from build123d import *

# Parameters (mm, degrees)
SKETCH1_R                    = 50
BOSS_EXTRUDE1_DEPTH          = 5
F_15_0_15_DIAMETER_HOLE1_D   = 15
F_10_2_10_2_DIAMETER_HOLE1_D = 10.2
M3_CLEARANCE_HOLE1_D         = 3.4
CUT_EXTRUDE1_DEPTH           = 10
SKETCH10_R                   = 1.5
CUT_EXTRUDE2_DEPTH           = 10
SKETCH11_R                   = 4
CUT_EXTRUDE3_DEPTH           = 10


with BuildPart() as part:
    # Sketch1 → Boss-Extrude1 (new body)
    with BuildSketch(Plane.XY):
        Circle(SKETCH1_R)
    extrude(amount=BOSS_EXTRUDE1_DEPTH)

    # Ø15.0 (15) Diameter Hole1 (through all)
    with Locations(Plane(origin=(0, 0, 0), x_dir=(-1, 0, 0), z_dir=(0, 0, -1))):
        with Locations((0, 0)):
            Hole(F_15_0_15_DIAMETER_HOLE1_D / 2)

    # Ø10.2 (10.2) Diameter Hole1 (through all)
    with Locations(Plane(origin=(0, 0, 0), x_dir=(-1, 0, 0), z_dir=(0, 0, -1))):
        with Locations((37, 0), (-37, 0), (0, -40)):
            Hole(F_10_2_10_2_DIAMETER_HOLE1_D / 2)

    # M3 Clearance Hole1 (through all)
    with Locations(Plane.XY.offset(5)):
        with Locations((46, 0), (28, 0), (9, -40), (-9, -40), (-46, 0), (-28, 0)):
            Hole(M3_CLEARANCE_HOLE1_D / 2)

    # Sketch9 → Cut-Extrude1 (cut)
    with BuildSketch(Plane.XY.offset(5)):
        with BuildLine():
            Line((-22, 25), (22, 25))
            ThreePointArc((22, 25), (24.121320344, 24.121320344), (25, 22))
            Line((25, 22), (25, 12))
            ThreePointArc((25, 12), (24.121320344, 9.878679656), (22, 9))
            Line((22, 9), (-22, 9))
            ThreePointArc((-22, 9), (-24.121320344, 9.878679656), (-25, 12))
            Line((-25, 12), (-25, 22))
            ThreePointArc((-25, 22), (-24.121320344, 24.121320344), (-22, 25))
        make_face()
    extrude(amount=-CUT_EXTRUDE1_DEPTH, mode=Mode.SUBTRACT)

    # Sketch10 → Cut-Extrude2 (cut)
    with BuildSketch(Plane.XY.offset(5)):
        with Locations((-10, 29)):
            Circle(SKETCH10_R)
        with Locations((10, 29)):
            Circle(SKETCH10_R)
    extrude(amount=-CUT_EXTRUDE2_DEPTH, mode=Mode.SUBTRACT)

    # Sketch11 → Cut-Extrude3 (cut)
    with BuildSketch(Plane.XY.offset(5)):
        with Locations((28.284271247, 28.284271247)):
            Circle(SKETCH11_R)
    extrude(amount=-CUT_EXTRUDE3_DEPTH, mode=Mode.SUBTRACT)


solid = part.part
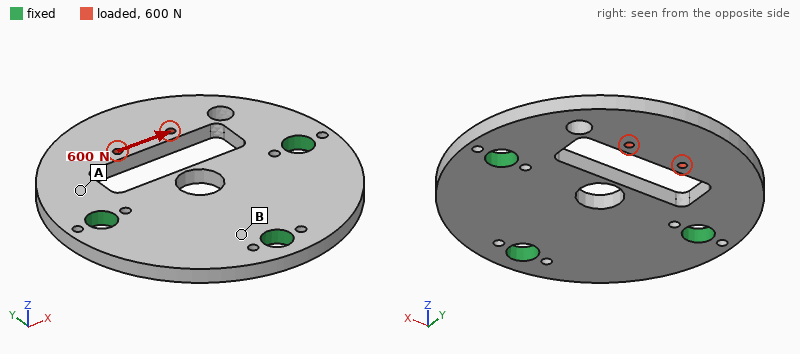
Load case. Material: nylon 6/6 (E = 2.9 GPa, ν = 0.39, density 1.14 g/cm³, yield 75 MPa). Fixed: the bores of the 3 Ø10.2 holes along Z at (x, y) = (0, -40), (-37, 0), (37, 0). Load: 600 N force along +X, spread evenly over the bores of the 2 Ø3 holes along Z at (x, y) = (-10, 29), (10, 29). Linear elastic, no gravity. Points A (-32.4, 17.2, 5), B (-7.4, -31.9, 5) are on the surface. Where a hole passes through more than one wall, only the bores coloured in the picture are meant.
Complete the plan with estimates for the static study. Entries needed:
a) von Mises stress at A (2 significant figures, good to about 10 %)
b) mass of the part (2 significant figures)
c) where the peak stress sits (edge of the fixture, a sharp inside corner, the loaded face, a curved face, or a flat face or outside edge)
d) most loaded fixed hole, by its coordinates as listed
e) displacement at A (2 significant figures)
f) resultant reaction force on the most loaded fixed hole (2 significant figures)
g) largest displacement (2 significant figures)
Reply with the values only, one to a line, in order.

7.5 MPa
37 g
a curved face
(-37, 0)
0.084 mm
360 N
0.25 mm
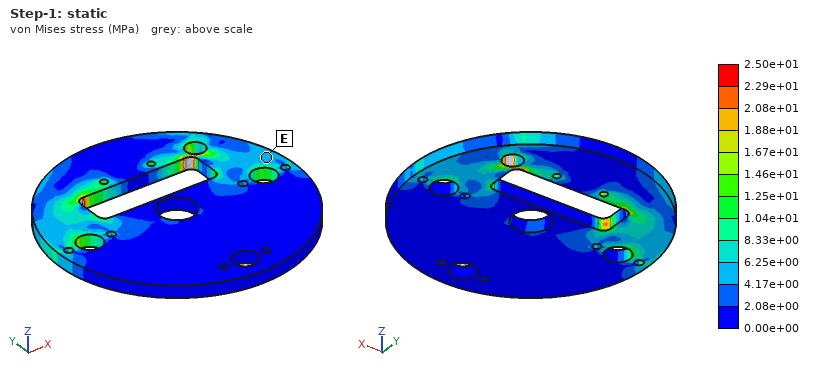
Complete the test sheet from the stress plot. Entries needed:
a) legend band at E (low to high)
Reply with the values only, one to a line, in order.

4.17e+00 to 6.25e+00 MPa
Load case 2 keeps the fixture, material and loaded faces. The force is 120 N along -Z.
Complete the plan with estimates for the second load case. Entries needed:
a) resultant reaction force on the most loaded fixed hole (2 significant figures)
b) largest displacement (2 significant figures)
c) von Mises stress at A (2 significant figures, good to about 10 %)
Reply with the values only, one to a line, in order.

65 N
1.6 mm
10 MPa
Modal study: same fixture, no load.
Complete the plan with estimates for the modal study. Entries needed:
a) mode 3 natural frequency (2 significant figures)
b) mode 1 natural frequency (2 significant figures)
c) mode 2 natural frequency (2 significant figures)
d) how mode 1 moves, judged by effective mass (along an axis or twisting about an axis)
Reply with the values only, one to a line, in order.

2100 Hz
510 Hz
1400 Hz
along Z
